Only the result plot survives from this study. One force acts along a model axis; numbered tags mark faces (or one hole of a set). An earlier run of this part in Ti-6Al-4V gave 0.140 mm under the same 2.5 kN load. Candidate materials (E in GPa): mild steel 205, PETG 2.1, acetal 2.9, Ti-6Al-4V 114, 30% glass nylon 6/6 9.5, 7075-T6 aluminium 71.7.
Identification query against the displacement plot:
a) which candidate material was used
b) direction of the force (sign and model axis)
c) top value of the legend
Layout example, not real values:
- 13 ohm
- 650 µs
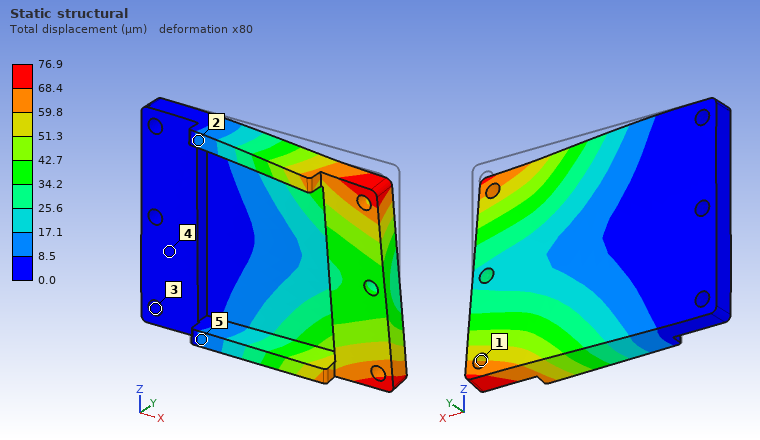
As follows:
- mild steel
- -Z
- 76.9 µm
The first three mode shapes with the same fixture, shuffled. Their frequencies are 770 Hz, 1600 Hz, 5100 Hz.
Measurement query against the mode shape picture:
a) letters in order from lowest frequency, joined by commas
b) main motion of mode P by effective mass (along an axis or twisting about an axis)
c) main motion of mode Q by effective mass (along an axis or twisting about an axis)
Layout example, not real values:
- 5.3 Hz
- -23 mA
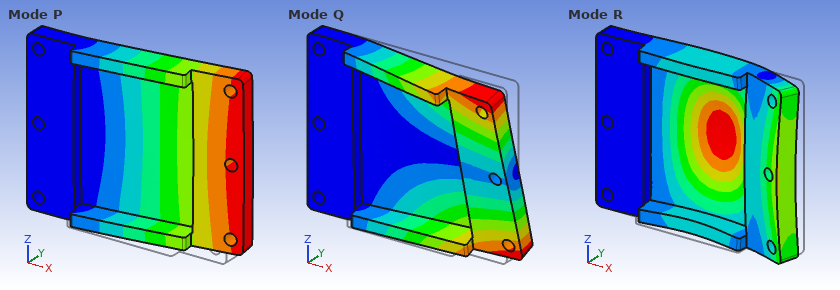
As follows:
- P, Q, R
- along Y
- twisting about X
